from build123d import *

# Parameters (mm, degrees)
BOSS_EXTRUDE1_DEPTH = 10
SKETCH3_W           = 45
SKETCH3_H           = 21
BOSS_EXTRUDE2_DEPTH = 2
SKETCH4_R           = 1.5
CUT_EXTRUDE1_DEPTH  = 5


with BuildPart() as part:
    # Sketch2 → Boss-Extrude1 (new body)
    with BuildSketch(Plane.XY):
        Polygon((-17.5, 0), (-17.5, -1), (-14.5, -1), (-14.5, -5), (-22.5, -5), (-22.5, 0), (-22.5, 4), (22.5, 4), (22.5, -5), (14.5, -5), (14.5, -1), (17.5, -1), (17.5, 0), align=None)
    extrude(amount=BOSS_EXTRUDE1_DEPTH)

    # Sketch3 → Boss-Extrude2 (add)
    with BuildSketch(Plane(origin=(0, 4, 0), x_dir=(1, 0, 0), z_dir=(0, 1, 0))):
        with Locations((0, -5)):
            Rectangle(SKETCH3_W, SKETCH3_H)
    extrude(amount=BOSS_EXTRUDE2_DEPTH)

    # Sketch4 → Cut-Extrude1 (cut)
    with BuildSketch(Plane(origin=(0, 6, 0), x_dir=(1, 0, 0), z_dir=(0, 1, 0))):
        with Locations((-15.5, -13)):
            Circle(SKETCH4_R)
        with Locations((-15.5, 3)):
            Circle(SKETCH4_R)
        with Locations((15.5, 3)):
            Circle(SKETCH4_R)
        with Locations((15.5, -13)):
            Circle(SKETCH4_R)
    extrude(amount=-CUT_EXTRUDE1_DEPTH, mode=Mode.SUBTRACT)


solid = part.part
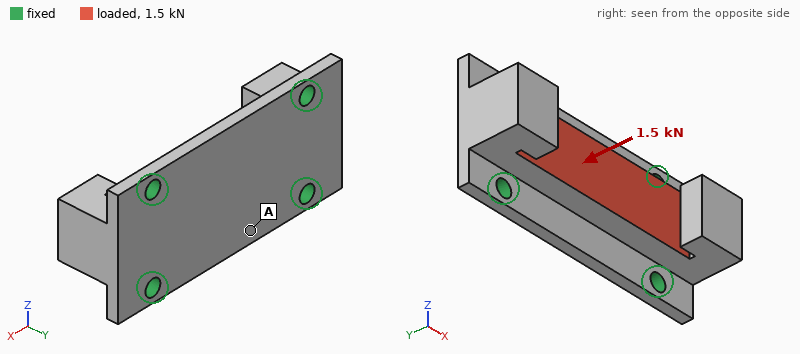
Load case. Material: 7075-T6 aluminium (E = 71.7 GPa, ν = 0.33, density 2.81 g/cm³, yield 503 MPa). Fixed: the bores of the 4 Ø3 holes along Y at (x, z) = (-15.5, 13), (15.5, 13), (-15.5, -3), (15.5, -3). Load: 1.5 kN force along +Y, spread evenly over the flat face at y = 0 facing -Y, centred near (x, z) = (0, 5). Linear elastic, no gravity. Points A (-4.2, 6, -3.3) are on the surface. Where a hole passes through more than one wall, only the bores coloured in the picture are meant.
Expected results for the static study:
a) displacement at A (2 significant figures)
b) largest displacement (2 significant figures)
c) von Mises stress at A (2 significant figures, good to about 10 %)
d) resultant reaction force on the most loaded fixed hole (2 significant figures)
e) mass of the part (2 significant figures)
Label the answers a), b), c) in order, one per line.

a) 21 µm
b) 23 µm
c) 25 MPa
d) 470 N
e) 12 g
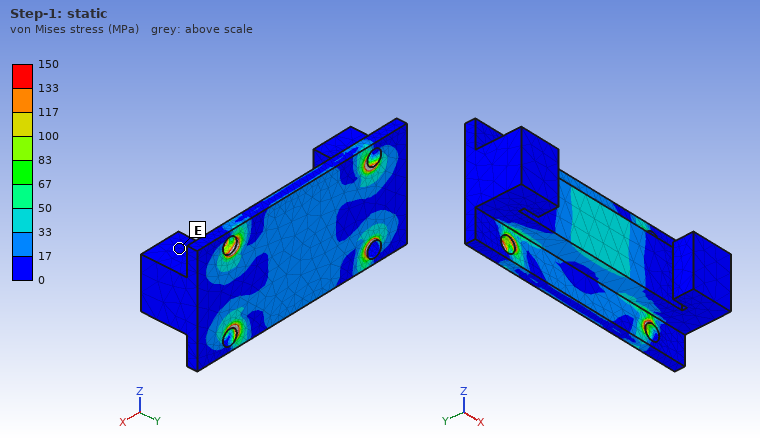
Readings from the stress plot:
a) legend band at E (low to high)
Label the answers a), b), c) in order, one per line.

a) 0 to 17 MPa
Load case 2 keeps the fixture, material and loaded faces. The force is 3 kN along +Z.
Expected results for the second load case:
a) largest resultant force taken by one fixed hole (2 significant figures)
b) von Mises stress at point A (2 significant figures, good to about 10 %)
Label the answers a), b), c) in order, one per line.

a) 1.0 kN
b) 29 MPa
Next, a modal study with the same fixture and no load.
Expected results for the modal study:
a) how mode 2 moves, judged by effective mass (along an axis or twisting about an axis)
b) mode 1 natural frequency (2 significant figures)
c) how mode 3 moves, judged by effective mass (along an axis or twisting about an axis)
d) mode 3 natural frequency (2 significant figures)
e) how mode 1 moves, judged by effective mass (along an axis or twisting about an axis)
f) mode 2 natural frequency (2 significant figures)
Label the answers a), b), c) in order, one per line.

a) along X
b) 15 kHz
c) along Y
d) 23 kHz
e) along Y
f) 20 kHz
